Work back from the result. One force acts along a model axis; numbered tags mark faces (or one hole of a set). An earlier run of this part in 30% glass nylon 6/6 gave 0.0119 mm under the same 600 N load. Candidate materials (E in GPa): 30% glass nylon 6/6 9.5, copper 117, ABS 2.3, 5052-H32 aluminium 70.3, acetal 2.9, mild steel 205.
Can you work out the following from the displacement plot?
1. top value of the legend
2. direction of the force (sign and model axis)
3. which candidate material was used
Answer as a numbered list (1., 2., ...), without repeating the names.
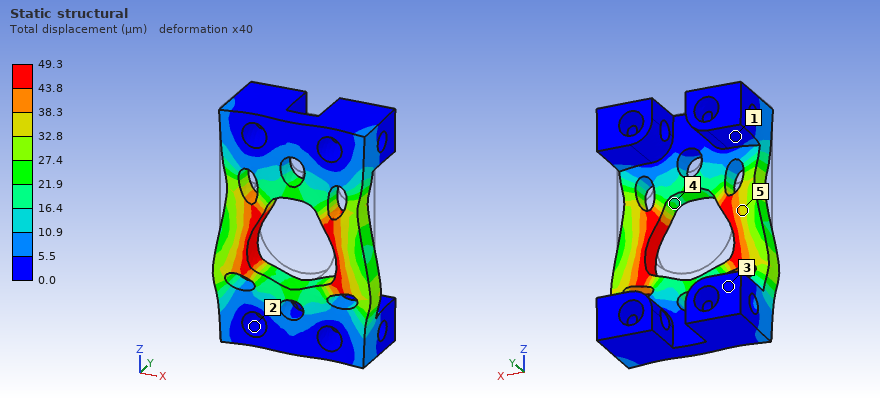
1. 49.3 µm
2. -Z
3. ABS
